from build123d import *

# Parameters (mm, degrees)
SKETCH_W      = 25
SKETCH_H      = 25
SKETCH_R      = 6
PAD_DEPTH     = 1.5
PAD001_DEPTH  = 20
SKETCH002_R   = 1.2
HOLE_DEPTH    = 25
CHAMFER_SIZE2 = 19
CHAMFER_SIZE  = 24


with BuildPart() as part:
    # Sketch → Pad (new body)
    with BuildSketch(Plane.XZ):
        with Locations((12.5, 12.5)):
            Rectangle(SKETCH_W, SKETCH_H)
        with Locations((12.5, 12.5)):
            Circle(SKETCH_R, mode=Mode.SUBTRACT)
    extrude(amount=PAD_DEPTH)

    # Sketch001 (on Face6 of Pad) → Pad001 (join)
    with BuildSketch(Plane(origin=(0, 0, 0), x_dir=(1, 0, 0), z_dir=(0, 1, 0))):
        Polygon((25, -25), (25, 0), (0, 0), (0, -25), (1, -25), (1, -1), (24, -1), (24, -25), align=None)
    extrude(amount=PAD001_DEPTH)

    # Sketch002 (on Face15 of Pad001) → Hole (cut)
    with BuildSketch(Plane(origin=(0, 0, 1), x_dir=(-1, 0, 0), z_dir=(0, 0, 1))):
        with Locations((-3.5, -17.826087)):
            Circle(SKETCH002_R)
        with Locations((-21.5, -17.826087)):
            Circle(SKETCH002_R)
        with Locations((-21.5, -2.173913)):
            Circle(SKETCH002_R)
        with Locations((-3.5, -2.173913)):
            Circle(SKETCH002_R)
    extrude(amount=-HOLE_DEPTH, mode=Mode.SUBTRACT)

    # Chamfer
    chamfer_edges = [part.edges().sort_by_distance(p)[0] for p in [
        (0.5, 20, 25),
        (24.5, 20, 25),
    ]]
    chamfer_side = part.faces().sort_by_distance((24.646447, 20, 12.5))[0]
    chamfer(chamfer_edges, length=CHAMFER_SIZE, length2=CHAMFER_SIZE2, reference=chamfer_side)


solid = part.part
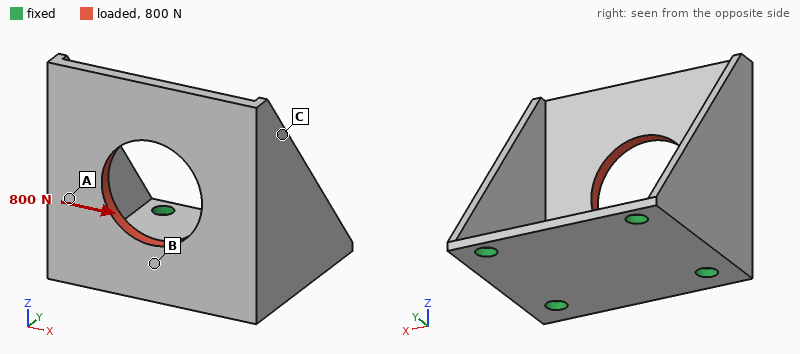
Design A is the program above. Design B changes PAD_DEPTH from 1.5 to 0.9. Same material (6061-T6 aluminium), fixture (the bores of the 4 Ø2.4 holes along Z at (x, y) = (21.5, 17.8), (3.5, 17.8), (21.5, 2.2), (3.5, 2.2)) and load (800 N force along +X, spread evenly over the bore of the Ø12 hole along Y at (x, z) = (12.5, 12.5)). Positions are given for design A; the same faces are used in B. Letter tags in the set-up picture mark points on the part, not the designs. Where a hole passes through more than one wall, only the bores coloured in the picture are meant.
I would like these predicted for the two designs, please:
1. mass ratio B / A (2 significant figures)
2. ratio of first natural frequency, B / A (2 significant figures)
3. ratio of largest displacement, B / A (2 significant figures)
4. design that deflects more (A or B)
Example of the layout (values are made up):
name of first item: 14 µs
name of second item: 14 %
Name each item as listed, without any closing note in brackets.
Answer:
mass ratio B / A: 0.82
ratio of first natural frequency, B / A: 0.82
ratio of largest displacement, B / A: 1.2
design that deflects more: B
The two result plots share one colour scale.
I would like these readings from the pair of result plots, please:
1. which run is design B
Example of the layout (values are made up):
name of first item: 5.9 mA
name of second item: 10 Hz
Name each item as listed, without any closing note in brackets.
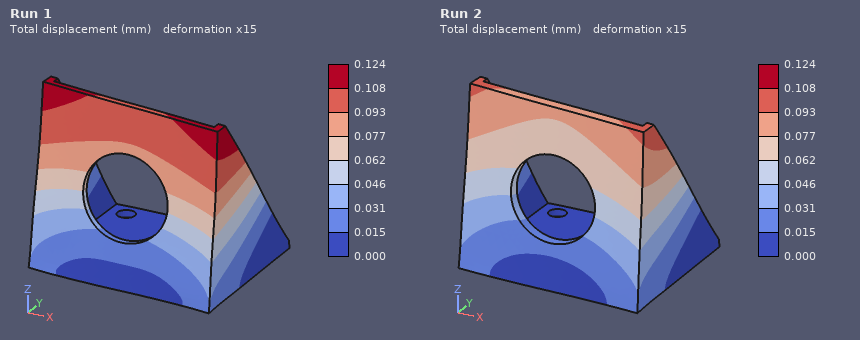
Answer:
which run is design B: Run 1
